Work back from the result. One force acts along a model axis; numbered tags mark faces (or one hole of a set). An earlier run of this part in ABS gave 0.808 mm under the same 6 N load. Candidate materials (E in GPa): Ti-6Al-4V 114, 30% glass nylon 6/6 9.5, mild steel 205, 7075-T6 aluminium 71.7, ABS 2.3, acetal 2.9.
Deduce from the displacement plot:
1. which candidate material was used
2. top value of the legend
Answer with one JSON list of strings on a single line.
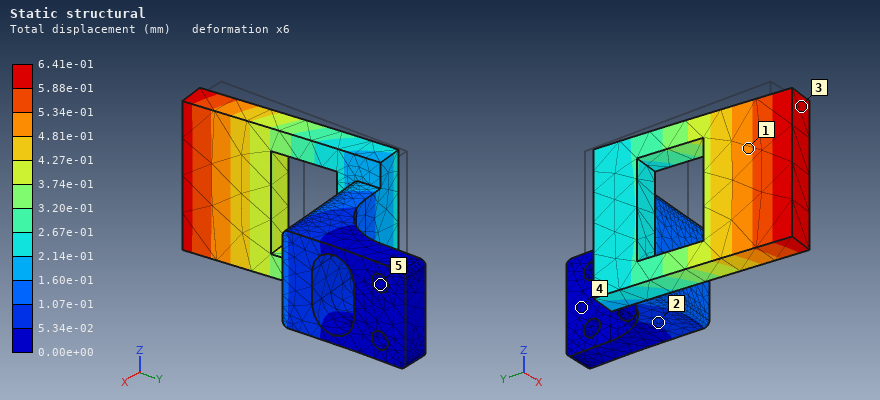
["acetal", "6.41e-01 mm"]
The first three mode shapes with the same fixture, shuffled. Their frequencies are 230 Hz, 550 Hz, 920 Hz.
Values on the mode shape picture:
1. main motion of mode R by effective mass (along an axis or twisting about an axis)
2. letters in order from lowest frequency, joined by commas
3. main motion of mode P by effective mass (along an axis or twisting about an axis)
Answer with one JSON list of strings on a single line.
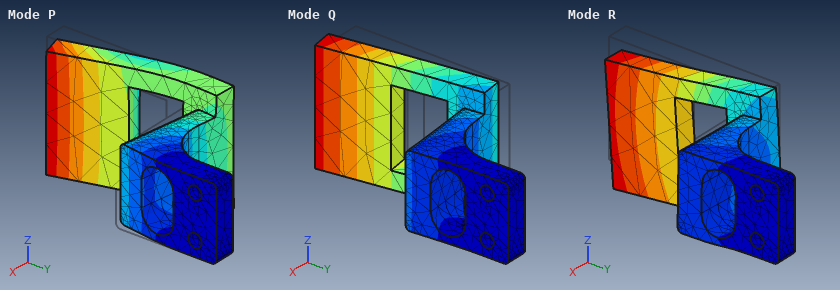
["along Z", "Q, R, P", "along Y"]
